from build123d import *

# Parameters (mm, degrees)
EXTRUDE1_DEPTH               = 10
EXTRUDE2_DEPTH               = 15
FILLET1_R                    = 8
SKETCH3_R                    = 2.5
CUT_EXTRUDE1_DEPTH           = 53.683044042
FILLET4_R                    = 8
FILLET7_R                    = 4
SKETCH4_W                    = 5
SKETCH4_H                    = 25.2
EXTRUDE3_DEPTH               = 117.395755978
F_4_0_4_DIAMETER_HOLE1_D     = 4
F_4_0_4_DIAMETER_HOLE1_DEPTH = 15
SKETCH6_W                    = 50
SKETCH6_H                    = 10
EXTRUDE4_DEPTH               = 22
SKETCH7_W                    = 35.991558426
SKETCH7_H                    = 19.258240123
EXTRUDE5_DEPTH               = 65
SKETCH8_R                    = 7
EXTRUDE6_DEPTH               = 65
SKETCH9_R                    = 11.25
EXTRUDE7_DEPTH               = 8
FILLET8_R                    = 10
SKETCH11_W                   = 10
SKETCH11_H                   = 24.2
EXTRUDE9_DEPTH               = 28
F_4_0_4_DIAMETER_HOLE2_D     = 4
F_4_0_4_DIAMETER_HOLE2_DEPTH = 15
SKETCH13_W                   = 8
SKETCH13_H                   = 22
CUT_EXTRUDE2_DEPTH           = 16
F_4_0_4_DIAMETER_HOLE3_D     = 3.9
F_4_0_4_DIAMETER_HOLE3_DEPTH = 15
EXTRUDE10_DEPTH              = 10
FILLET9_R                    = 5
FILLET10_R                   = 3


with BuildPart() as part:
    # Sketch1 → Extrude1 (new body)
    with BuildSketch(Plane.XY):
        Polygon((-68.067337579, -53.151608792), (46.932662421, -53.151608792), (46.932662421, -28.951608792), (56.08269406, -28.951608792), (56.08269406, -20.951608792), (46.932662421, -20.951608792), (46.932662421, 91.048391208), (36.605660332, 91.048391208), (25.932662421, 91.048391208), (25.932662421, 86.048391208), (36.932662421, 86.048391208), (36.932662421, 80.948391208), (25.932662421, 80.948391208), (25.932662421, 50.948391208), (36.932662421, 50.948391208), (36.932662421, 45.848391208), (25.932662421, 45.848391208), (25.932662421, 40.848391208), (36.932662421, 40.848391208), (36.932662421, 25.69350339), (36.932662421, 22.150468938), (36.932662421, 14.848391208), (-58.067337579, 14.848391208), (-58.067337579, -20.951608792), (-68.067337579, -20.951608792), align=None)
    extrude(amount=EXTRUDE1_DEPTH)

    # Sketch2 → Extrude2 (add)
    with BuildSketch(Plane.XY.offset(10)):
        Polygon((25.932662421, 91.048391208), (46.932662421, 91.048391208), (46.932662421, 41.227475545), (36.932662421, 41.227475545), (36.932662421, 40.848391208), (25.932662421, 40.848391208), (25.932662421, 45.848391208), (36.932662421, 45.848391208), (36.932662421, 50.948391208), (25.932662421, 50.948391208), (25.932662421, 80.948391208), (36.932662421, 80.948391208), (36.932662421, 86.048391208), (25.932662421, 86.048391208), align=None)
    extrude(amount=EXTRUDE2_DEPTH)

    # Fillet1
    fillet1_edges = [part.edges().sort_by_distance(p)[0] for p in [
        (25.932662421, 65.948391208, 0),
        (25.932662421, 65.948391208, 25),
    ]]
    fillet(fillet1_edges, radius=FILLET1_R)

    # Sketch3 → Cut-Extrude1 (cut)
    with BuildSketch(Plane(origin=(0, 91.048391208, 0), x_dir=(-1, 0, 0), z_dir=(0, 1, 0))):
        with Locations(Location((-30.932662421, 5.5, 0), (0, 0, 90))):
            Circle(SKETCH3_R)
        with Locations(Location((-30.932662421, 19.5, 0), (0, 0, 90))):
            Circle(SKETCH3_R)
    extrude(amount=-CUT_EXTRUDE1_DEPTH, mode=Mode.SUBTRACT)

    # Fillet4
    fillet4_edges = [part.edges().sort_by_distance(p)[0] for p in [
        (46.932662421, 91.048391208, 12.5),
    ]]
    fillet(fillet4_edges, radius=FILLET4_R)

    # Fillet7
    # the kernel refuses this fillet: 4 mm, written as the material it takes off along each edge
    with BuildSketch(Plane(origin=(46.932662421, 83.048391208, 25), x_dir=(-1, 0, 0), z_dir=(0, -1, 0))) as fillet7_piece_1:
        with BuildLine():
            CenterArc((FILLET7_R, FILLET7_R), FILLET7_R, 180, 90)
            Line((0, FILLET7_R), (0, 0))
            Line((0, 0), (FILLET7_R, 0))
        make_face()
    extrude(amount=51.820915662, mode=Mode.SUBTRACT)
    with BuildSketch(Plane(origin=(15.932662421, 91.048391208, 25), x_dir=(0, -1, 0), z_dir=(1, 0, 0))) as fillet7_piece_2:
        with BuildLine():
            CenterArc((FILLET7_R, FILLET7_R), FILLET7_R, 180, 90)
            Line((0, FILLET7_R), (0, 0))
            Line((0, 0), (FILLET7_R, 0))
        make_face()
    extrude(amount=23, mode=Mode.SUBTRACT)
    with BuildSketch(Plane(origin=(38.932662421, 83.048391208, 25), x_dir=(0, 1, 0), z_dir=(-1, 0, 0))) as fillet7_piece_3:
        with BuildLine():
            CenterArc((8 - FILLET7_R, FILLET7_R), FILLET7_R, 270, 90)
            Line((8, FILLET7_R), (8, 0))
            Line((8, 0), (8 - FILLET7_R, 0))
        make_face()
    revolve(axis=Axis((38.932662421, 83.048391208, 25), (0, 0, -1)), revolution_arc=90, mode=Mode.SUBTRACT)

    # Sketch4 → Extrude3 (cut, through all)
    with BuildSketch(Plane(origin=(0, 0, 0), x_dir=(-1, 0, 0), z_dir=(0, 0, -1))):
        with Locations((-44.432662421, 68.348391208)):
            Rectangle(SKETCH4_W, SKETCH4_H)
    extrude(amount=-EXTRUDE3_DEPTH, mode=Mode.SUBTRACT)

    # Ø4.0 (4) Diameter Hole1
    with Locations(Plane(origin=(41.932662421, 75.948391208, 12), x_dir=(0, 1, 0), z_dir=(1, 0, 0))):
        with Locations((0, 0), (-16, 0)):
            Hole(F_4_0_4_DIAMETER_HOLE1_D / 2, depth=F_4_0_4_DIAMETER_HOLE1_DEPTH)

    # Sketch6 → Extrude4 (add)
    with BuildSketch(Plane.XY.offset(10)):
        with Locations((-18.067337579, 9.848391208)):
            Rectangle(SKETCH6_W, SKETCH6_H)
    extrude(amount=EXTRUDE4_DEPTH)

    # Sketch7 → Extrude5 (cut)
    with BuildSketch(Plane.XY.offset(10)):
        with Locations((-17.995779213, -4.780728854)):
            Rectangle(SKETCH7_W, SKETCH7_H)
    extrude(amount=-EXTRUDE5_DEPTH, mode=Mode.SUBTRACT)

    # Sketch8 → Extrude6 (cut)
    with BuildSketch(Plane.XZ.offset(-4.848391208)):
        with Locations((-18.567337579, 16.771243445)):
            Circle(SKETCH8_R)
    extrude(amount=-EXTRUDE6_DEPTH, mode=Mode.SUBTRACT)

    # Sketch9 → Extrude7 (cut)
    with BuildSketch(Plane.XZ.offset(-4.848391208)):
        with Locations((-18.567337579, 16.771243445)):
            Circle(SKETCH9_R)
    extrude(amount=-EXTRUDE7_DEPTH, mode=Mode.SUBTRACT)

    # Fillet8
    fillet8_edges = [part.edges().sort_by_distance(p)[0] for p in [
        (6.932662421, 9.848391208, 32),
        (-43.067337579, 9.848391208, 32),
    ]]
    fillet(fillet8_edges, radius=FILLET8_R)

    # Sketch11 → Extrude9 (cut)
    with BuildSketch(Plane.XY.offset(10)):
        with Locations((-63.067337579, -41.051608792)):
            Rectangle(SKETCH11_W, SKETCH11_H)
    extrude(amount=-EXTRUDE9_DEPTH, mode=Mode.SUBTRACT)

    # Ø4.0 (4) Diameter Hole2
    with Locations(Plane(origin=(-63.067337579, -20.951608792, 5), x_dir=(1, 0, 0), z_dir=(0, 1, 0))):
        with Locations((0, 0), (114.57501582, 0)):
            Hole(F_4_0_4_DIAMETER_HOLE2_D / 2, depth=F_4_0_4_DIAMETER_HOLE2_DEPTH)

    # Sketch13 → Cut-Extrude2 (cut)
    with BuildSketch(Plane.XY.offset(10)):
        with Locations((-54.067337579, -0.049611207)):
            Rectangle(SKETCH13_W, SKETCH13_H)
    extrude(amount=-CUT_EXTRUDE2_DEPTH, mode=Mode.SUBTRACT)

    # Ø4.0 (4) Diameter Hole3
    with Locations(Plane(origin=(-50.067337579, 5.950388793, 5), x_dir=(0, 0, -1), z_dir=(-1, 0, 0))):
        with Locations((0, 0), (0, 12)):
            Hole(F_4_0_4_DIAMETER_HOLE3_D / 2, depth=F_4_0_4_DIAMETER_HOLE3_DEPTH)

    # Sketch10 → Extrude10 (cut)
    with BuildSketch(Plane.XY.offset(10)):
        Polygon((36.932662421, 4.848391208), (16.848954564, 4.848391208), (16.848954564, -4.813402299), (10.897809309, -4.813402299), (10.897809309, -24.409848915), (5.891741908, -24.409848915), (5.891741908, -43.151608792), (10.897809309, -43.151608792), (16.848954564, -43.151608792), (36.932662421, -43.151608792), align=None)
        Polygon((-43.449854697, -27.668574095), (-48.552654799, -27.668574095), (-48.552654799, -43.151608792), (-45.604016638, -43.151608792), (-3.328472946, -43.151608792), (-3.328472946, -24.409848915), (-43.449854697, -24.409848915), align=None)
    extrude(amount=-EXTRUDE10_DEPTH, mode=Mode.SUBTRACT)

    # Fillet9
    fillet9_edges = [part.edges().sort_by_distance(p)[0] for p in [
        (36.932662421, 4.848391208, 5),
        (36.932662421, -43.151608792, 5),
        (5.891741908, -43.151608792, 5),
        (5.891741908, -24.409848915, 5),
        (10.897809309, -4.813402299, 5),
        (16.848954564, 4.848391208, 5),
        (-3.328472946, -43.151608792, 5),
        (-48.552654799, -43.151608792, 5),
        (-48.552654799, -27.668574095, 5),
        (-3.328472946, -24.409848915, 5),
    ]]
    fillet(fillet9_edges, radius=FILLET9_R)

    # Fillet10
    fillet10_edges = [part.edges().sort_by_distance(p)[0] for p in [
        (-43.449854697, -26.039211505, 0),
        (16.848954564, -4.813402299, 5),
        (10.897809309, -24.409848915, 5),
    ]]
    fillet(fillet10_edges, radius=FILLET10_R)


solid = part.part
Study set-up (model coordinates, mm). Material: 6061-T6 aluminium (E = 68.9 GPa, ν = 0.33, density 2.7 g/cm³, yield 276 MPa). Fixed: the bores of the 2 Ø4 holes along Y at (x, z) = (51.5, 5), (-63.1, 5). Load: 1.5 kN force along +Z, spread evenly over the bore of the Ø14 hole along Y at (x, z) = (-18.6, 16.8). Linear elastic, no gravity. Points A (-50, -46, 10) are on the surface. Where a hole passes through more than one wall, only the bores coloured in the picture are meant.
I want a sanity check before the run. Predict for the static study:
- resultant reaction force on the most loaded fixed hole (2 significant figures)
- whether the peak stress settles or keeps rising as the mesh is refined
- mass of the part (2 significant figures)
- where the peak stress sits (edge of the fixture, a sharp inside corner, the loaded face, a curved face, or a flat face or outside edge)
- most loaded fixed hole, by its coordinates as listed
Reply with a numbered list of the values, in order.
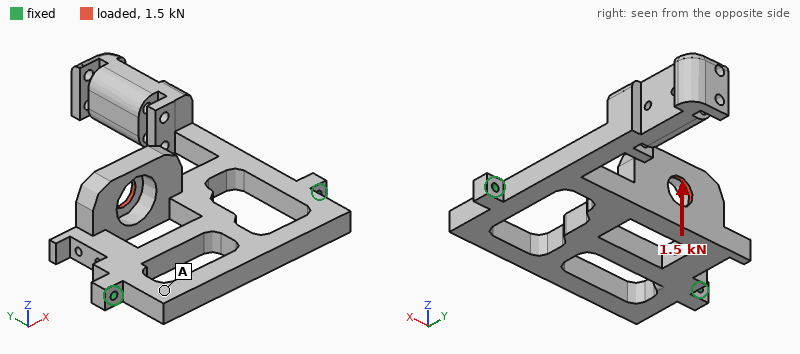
1. 960 N
2. keeps rising
3. 190 g
4. edge of the fixture
5. (-63.1, 5)
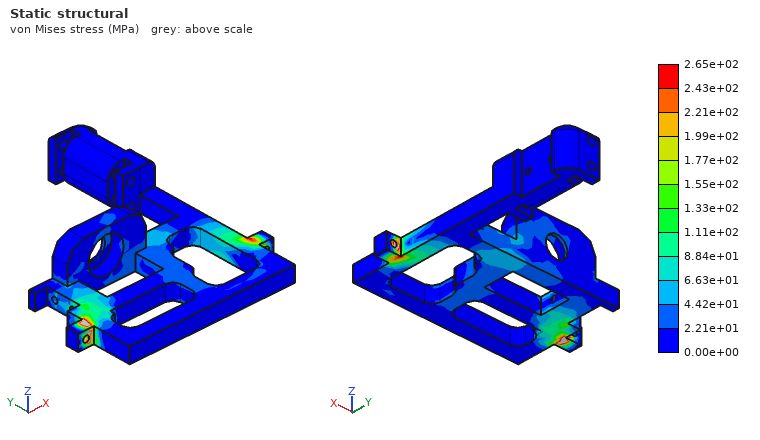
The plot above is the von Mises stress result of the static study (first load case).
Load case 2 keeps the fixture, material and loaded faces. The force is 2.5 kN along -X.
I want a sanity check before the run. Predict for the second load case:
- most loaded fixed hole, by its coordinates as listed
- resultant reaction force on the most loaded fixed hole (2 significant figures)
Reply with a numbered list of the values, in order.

1. (-63.1, 5)
2. 2.1 kN
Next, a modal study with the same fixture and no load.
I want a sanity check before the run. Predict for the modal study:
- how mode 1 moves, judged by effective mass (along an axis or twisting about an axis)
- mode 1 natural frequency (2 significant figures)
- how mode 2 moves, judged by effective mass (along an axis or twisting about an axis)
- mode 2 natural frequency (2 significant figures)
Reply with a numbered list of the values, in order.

1. along Z
2. 350 Hz
3. along X
4. 610 Hz
